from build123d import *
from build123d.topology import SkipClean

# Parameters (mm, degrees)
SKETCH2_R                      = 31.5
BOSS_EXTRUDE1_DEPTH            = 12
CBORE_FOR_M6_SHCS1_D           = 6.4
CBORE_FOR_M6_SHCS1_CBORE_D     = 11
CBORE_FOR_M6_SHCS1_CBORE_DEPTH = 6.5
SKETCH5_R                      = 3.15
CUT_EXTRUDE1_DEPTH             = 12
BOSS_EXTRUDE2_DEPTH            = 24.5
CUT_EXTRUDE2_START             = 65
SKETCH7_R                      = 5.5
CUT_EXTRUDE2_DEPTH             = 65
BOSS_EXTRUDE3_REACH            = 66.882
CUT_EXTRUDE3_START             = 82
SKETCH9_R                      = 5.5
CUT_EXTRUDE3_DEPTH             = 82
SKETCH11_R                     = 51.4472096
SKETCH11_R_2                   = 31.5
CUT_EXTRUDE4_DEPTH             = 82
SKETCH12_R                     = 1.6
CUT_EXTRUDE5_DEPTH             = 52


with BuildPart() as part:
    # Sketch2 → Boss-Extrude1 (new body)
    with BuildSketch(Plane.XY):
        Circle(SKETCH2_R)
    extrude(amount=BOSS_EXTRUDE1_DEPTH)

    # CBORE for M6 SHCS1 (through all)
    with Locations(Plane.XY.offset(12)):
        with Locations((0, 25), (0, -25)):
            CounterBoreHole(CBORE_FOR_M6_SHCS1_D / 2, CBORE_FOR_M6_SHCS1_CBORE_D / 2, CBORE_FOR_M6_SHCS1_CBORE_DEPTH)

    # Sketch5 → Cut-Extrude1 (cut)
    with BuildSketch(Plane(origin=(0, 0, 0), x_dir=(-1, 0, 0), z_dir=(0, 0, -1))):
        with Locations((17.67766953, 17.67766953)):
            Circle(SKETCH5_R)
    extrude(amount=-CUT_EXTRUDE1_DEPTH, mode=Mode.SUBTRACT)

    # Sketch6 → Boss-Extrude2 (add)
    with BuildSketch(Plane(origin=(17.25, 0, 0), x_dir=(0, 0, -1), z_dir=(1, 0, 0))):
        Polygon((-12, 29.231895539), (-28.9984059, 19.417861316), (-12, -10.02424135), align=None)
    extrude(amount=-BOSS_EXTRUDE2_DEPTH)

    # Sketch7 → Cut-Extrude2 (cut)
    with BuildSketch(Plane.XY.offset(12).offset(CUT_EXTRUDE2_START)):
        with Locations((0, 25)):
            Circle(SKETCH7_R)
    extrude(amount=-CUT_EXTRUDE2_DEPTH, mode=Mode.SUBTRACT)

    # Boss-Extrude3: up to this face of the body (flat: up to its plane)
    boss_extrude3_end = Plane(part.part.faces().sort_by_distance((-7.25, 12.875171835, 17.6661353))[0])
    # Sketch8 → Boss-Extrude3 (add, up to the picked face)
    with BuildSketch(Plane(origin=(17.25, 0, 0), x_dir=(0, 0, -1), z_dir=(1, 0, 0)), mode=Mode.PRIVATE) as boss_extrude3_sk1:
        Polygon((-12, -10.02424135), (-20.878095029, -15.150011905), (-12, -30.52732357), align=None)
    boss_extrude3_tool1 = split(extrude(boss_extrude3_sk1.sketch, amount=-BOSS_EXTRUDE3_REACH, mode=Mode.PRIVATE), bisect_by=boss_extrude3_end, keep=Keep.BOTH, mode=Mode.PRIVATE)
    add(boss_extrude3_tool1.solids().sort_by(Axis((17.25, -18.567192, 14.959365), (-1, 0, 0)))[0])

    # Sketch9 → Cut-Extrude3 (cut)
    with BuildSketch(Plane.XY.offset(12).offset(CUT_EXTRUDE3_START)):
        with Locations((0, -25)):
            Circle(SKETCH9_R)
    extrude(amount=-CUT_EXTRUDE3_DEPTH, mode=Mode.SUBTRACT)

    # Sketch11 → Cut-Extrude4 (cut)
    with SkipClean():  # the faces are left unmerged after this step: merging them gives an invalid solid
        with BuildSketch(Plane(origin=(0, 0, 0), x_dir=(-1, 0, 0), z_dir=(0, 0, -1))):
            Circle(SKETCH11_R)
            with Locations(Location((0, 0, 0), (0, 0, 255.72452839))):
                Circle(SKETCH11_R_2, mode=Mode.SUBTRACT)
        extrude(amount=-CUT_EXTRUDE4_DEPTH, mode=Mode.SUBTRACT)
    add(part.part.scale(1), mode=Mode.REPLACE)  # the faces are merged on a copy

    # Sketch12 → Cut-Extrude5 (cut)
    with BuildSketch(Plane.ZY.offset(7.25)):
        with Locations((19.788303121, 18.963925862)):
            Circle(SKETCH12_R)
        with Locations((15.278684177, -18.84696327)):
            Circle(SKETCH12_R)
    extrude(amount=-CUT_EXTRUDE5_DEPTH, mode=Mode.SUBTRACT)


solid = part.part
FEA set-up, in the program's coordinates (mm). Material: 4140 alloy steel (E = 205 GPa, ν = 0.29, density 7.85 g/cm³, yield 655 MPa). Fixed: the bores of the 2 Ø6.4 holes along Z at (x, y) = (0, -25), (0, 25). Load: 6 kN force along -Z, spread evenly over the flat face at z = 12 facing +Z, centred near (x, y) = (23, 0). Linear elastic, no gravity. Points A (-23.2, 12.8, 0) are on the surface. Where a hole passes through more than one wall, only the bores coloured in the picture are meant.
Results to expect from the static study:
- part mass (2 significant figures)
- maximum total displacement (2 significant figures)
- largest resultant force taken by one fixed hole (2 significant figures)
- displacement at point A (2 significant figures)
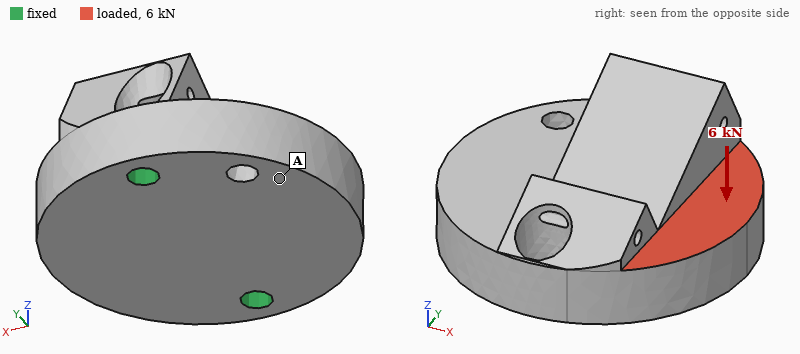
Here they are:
350 g
85 µm
3.6 kN
43 µm
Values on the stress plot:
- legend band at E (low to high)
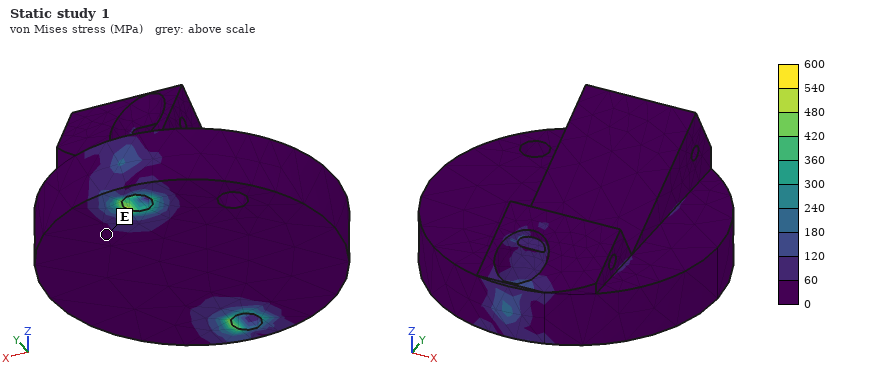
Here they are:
0 to 60 MPa
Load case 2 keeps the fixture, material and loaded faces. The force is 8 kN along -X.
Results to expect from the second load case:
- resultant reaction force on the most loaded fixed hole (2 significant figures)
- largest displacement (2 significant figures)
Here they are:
4.0 kN
46 µm
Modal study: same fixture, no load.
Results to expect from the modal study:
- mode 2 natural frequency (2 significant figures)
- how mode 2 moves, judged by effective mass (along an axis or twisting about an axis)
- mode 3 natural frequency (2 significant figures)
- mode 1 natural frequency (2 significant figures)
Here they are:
9400 Hz
along Z
16 kHz
4100 Hz
